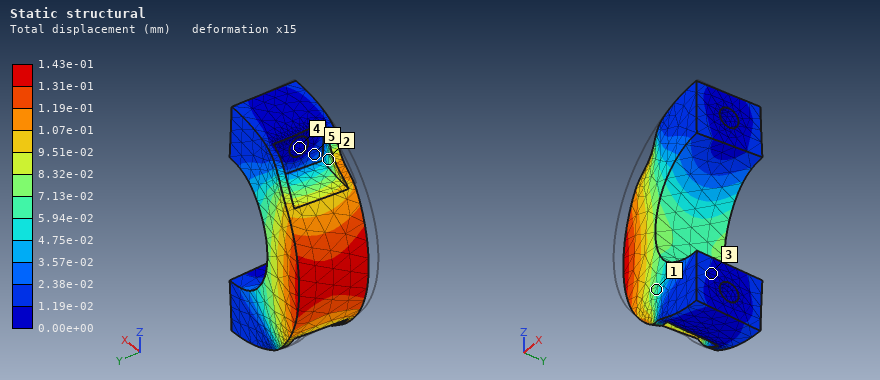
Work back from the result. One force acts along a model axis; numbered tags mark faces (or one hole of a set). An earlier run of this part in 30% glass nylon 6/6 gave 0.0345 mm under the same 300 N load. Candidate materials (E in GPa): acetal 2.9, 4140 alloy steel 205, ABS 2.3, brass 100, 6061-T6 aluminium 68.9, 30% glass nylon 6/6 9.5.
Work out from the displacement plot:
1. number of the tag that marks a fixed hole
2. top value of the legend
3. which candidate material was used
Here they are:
4
1.43e-01 mm
ABS
